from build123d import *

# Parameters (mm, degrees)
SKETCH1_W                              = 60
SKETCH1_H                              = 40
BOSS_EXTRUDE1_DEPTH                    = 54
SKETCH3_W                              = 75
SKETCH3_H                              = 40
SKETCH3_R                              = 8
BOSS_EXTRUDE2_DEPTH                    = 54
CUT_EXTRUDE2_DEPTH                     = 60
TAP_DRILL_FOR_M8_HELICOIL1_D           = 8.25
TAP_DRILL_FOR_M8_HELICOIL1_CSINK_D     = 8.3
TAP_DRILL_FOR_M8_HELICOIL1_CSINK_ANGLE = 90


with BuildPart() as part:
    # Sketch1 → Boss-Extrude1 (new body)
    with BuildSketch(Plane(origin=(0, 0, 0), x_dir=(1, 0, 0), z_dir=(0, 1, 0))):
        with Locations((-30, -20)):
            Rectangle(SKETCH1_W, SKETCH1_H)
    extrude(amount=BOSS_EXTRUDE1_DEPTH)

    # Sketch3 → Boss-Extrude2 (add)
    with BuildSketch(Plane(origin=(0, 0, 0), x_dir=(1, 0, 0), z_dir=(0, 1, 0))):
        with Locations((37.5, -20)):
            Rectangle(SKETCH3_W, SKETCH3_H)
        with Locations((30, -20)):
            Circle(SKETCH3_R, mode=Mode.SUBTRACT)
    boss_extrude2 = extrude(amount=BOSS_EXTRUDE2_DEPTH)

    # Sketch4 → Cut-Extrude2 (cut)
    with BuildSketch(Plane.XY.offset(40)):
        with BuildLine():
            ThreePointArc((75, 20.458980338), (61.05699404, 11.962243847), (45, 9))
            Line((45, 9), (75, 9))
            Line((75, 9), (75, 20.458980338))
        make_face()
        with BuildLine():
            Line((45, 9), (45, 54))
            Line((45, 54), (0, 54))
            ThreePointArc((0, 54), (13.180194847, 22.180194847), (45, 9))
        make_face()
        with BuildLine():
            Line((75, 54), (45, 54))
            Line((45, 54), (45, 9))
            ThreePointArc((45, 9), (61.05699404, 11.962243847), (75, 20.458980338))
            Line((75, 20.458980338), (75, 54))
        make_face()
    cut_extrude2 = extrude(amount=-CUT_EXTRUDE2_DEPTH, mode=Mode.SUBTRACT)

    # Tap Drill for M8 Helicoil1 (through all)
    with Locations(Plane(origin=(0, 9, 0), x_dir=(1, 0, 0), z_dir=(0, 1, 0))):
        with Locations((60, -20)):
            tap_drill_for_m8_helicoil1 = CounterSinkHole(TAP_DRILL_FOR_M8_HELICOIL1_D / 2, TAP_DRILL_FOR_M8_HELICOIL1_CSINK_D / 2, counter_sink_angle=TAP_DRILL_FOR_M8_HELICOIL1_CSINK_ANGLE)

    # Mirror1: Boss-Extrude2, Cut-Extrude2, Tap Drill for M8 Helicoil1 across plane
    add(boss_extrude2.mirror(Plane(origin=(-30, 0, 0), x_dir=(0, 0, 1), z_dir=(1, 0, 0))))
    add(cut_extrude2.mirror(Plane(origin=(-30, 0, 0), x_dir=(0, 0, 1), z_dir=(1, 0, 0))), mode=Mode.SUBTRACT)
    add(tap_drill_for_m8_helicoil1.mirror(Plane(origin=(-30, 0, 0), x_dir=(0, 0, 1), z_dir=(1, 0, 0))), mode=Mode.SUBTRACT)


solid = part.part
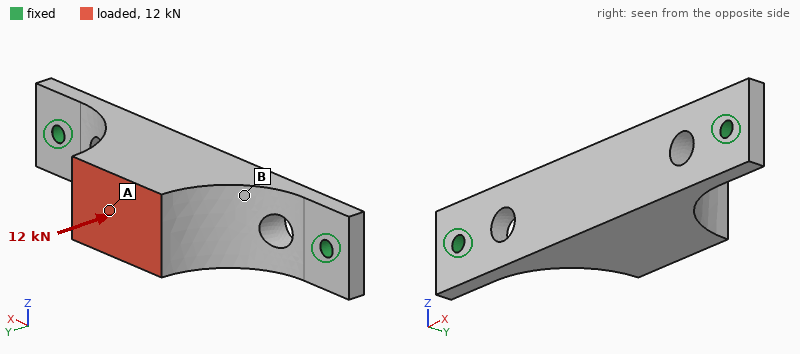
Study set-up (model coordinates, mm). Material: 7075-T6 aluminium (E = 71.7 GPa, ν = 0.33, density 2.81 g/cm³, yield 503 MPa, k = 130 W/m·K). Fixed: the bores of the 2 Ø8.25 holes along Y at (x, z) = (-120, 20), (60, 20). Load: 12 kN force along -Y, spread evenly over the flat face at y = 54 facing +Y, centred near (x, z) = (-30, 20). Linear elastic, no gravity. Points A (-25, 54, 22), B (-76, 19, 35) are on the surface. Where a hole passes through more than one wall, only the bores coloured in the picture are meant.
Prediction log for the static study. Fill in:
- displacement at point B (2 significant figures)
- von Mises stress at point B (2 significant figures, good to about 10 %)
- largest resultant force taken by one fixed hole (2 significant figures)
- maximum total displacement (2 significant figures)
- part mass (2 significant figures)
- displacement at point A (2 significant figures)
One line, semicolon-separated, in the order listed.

0.21 mm; 75 MPa; 8.9 kN; 0.22 mm; 600 g; 0.22 mm
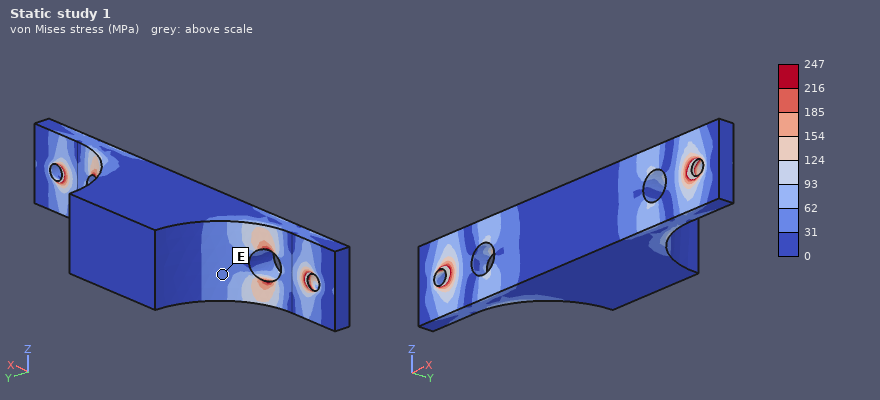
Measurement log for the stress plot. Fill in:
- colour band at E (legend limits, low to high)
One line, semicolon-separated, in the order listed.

31 to 62 MPa
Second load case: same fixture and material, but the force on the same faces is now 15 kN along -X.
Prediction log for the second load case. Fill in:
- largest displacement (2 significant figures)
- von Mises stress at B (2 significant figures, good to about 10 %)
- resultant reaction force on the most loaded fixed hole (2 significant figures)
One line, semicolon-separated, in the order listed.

0.15 mm; 67 MPa; 9.0 kN
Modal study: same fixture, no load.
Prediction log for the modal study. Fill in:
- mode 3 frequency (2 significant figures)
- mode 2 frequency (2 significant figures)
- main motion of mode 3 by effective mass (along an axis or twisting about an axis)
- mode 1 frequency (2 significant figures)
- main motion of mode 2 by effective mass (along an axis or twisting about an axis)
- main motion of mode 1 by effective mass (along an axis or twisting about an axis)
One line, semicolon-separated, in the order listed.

3200 Hz; 1600 Hz; along Z; 940 Hz; along Y; along Z
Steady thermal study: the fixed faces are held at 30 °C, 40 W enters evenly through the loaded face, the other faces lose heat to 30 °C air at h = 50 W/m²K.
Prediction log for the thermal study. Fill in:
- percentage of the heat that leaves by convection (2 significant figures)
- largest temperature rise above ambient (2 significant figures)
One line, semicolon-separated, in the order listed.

40 %; 20 K
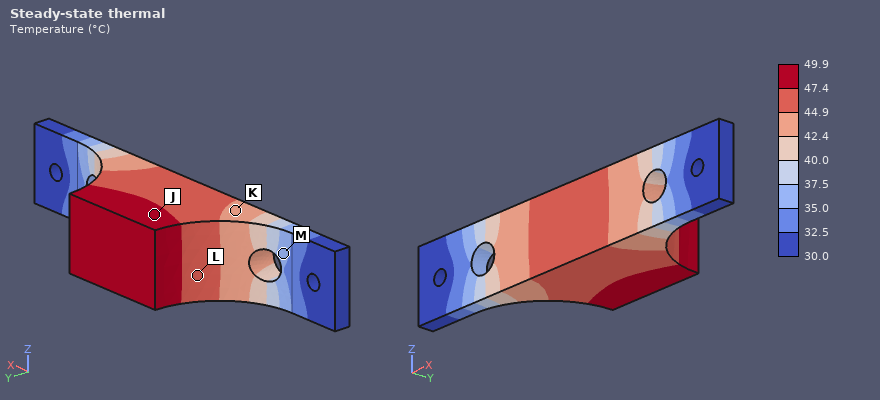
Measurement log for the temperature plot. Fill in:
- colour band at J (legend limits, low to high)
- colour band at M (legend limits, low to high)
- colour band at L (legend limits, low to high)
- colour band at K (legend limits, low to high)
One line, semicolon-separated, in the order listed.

47.4 to 49.9 °C; 35.0 to 37.5 °C; 44.9 to 47.4 °C; 42.4 to 44.9 °C
